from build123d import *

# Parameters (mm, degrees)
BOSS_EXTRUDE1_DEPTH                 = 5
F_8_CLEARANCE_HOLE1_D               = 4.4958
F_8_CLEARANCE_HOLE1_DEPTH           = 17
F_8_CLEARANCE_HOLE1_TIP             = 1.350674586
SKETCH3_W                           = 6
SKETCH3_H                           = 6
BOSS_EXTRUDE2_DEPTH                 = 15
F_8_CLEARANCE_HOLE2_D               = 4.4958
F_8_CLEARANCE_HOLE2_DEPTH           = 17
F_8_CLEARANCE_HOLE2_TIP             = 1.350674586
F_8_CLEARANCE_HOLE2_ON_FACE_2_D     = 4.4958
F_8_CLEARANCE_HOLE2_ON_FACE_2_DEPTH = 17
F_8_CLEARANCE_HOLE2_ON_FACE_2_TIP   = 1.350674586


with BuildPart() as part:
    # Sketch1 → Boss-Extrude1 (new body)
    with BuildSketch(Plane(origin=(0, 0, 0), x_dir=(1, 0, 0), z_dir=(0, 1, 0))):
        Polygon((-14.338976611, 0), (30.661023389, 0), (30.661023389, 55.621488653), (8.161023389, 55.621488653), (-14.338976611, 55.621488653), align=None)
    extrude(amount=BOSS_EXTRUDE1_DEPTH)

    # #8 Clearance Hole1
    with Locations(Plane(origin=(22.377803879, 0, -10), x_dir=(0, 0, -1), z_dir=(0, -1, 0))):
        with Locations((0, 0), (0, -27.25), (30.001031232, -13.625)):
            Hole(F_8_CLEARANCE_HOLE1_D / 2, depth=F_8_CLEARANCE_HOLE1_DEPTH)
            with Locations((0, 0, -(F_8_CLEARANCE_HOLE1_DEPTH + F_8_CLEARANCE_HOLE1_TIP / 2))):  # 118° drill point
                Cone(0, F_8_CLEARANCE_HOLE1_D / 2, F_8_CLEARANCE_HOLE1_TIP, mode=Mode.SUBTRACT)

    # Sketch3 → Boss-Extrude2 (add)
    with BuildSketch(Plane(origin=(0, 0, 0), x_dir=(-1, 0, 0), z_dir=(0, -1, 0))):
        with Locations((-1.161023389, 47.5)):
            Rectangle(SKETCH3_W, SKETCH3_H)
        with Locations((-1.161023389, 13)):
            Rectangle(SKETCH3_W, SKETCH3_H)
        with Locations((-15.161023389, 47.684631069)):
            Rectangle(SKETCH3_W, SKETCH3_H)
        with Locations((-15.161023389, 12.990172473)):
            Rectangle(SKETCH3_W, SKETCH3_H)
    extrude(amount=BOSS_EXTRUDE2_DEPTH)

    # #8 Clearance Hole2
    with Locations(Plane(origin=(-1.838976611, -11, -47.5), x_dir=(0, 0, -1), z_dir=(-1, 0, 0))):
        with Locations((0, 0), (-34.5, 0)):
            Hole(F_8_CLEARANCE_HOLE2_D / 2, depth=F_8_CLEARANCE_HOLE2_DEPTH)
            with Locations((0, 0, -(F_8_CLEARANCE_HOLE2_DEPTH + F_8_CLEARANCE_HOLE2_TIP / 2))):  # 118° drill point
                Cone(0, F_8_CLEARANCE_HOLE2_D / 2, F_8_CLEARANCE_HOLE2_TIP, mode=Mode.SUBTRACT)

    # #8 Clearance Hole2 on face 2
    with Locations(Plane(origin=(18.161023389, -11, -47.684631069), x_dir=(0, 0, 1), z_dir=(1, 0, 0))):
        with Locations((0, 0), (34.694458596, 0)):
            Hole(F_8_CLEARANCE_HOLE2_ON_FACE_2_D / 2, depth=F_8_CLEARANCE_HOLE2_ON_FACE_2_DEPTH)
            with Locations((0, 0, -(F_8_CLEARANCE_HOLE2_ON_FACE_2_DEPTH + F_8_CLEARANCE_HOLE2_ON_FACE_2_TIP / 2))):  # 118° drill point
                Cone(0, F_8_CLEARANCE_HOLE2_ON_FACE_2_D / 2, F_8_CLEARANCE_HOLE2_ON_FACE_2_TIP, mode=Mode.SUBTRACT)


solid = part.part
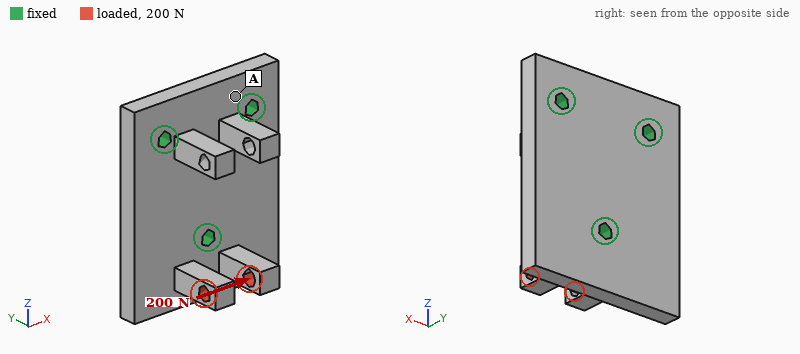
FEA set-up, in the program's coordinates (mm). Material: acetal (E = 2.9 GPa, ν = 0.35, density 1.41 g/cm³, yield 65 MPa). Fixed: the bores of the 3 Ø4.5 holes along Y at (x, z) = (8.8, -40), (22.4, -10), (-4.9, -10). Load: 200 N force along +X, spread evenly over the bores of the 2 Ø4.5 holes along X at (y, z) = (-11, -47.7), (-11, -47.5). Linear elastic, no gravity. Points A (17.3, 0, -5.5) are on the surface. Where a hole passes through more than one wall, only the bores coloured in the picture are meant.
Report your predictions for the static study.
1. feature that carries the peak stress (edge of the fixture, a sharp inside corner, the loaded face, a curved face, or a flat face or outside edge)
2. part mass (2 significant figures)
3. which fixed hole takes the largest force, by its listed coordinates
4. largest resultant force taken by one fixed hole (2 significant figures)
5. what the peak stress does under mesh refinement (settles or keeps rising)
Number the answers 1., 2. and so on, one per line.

1. edge of the fixture
2. 20 g
3. (8.8, -40)
4. 210 N
5. keeps rising
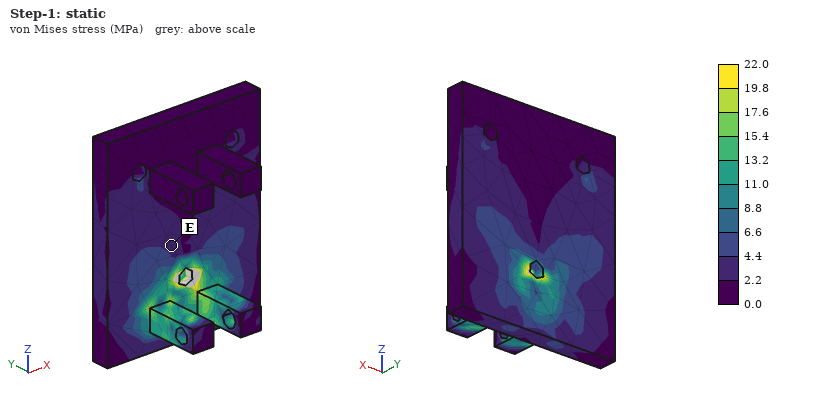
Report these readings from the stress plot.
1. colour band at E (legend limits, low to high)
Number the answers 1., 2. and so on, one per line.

1. 2.2 to 4.4 MPa
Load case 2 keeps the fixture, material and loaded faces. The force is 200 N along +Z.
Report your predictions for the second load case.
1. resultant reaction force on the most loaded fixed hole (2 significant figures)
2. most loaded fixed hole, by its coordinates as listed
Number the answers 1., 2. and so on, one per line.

1. 150 N
2. (8.8, -40)
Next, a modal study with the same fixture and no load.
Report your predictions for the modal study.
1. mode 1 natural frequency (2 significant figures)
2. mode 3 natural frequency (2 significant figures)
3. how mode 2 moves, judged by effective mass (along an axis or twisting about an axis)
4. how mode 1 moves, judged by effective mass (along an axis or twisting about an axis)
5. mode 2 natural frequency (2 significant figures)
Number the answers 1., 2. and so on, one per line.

1. 2000 Hz
2. 3300 Hz
3. along Y
4. twisting about Z
5. 2400 Hz
